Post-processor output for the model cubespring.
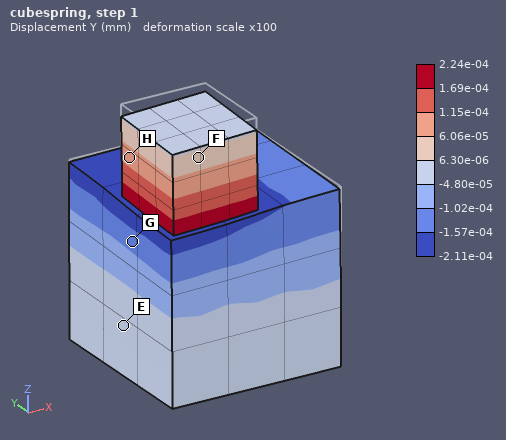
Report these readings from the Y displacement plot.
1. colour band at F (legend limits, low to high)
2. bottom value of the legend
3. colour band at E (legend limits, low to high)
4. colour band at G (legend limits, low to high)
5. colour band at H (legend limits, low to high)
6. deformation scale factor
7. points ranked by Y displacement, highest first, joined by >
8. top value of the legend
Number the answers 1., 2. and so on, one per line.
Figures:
1. 6.30e-06 to 6.06e-05 mm
2. -2.11e-04 mm
3. -4.80e-05 to 6.30e-06 mm
4. -1.57e-04 to -1.02e-04 mm
5. 6.06e-05 to 1.15e-04 mm
6. 100
7. H > F > E > G
8. 2.24e-04 mm
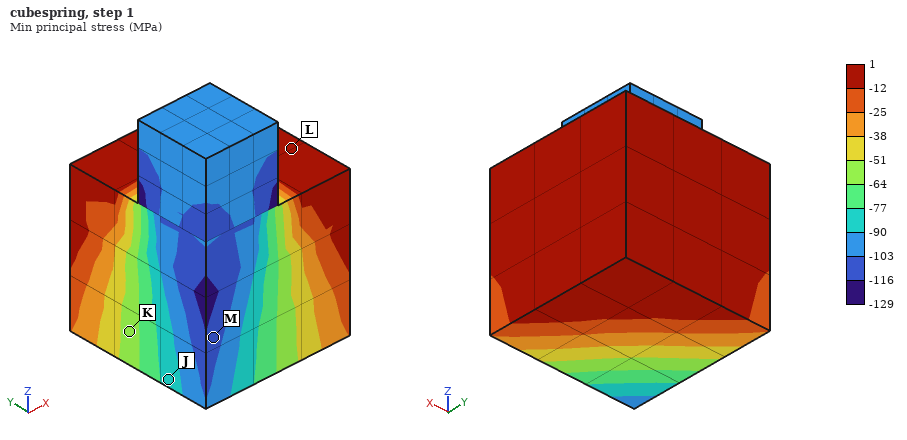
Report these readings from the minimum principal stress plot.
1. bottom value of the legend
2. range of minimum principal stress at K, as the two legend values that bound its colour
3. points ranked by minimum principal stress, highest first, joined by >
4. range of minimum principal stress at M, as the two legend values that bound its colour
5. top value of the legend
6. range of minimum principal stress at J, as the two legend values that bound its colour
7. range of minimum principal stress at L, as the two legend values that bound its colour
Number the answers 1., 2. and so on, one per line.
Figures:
1. -129 MPa
2. -64 to -51 MPa
3. L > K > J > M
4. -116 to -103 MPa
5. 1 MPa
6. -90 to -77 MPa
7. -12 to 1 MPa
